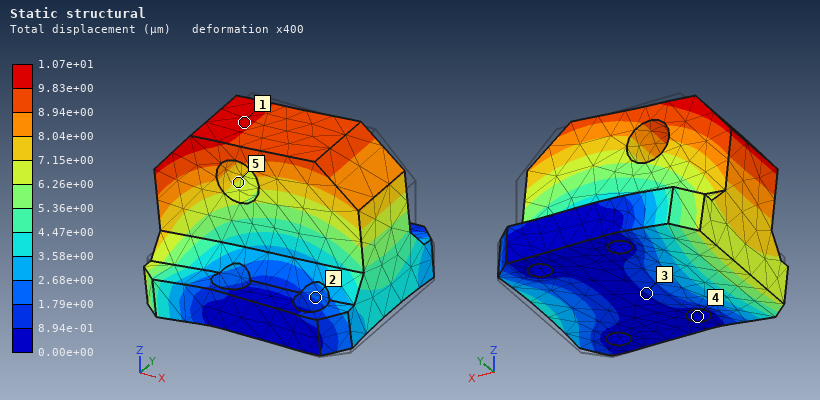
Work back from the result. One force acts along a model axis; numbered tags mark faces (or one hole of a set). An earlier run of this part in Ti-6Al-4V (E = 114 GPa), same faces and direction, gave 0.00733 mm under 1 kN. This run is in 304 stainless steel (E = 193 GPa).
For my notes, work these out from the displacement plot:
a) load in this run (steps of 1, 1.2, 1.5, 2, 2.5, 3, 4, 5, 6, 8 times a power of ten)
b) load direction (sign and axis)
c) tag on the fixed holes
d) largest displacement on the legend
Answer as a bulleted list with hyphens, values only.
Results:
- 2.5 kN
- -X
- 4
- 1.07e+01 µm
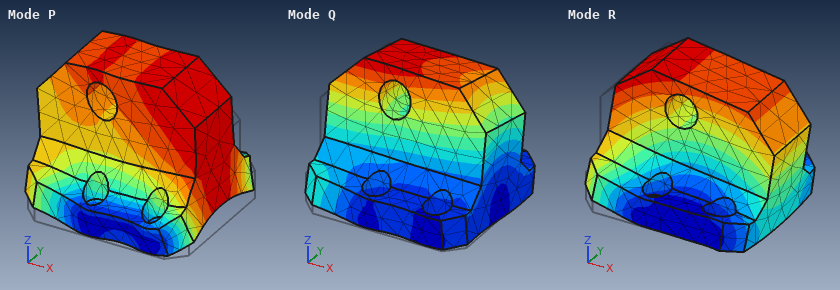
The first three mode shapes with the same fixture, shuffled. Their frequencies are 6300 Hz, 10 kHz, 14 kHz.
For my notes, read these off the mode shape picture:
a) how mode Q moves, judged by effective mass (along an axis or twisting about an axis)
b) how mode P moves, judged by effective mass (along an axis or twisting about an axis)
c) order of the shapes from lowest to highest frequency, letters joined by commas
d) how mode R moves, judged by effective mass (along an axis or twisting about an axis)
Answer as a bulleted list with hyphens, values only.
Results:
- along Y
- along Z
- R, Q, P
- along X
